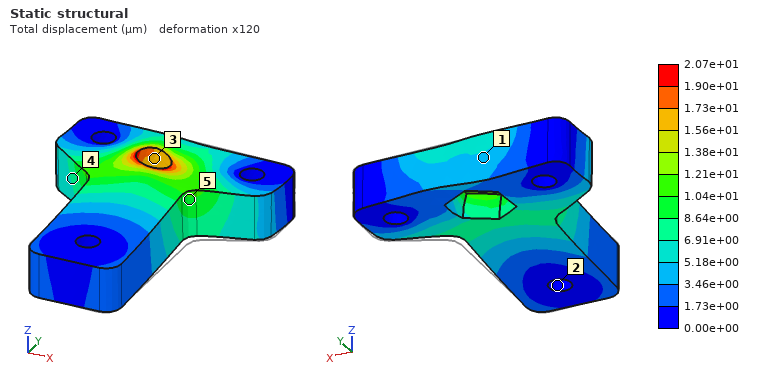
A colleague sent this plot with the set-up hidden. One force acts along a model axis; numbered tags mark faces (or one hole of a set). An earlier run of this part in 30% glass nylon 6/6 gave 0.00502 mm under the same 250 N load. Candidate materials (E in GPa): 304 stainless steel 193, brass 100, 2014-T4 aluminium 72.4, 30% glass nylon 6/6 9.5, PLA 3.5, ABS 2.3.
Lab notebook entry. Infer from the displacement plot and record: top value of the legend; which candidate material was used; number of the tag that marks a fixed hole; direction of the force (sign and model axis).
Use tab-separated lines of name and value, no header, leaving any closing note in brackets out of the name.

top value of the legend	2.07e+01 µm
which candidate material was used	ABS
number of the tag that marks a fixed hole	2
direction of the force	-X
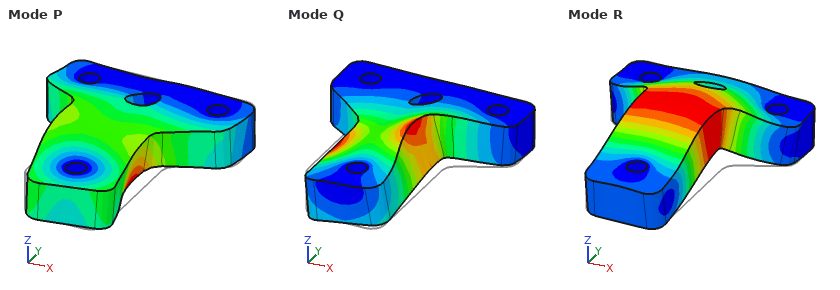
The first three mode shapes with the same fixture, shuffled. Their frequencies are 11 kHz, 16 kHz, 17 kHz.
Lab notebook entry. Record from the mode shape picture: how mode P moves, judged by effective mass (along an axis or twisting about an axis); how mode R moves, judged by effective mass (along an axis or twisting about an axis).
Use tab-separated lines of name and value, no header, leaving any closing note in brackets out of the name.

how mode P moves, judged by effective mass	along X
how mode R moves, judged by effective mass	along Z
